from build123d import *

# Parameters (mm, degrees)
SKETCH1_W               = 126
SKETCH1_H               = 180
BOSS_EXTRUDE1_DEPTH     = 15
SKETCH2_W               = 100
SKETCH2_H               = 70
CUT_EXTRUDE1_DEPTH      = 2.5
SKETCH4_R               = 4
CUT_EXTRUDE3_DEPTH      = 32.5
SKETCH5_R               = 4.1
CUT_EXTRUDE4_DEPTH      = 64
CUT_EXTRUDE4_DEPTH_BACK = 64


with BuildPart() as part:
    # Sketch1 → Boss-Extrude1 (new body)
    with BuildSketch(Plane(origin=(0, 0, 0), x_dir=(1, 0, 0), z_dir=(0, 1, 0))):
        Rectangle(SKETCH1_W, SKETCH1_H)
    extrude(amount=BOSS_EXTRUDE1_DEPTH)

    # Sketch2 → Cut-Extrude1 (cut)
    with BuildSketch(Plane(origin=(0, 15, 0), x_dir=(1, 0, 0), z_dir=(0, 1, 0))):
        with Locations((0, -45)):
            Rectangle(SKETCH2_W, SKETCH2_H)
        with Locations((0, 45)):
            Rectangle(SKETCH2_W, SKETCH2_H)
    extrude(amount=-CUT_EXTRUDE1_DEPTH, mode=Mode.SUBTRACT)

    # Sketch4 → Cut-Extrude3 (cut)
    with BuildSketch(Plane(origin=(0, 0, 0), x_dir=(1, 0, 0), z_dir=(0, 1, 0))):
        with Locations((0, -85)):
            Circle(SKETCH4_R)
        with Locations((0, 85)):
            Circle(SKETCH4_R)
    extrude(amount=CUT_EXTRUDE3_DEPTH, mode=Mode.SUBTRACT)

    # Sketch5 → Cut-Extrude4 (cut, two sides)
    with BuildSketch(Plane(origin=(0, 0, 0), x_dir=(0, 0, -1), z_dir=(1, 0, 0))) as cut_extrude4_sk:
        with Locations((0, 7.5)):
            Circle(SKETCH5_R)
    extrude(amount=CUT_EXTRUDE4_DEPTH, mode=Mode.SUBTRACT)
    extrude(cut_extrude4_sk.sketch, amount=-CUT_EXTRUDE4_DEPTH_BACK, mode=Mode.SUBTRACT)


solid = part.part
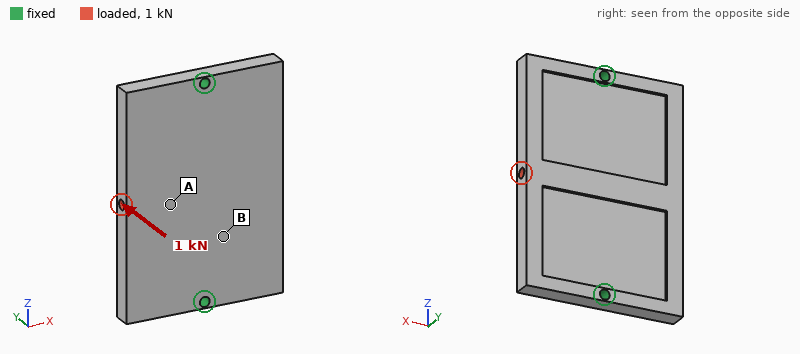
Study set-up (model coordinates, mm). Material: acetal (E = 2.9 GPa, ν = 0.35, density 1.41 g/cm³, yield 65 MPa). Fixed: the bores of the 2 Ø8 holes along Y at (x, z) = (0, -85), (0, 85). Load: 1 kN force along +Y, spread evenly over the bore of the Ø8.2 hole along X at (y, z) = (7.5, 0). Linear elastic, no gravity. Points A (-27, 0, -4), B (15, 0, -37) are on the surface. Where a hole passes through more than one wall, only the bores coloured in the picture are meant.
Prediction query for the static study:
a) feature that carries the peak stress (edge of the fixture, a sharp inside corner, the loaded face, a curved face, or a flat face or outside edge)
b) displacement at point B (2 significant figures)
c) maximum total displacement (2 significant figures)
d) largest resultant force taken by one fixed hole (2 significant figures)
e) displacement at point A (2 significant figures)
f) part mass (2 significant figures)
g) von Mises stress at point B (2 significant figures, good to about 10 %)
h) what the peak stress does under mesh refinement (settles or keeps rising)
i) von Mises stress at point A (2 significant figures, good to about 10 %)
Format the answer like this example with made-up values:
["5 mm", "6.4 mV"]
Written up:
["edge of the fixture", "0.47 mm", "0.84 mm", "500 N", "0.69 mm", "420 g", "3.0 MPa", "keeps rising", "6.0 MPa"]
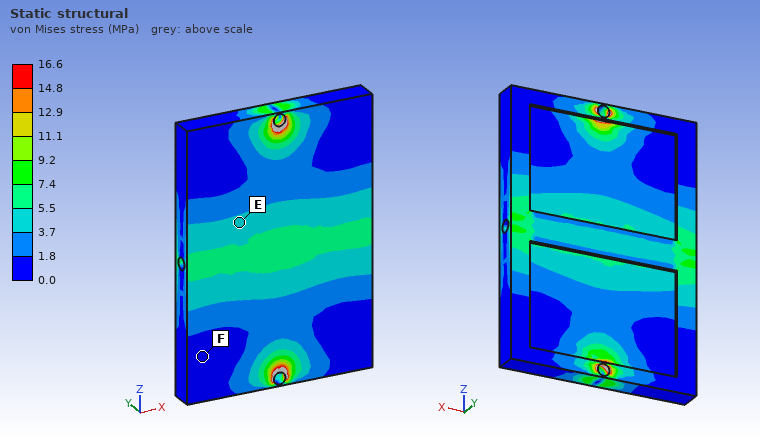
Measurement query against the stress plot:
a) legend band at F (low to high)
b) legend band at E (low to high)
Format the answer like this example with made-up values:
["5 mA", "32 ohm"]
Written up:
["0.0 to 1.8 MPa", "3.7 to 5.5 MPa"]
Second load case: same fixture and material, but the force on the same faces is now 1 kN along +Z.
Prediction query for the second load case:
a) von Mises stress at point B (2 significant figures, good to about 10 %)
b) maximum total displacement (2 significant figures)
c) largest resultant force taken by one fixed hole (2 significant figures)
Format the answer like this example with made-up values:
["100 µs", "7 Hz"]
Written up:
["0.46 MPa", "24 µm", "500 N"]
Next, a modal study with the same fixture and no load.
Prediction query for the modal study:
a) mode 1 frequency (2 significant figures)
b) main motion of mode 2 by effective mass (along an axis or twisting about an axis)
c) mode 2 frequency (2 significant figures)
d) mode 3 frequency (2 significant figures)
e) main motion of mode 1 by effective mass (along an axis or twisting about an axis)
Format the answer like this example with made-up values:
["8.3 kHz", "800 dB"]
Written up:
["350 Hz", "along Y", "420 Hz", "790 Hz", "twisting about Z"]
